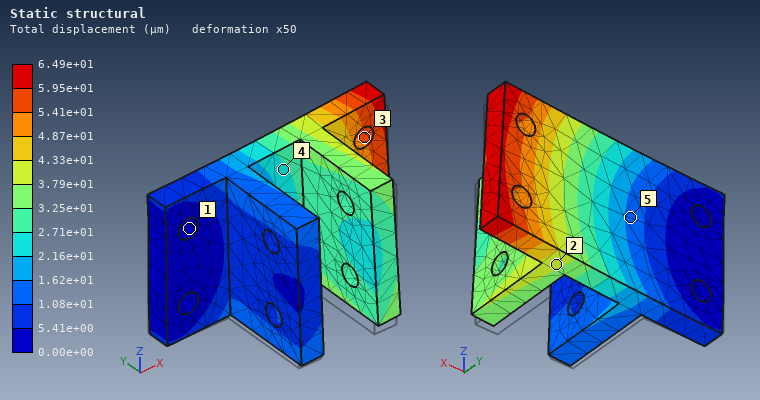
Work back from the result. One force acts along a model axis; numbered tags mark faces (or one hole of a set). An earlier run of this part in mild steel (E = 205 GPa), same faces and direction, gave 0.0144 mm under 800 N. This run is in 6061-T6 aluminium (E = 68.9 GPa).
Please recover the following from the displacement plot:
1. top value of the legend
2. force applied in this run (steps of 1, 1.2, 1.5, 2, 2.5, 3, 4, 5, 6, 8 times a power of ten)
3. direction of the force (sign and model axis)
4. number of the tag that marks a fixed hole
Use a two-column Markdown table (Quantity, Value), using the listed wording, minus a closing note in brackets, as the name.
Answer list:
| Quantity | Value |
|---|---|
| top value of the legend | 6.49e+01 µm |
| force applied in this run | 1.2 kN |
| direction of the force | +Z |
| number of the tag that marks a fixed hole | 1 |
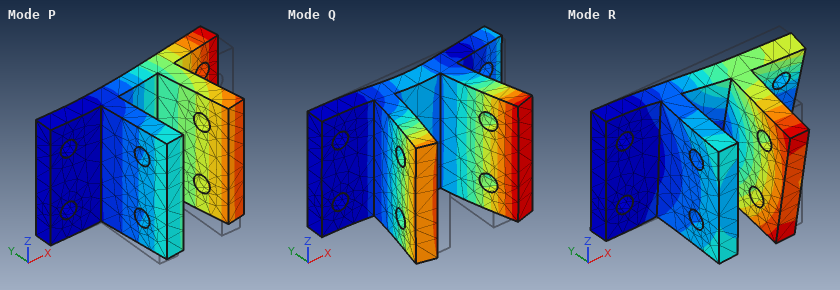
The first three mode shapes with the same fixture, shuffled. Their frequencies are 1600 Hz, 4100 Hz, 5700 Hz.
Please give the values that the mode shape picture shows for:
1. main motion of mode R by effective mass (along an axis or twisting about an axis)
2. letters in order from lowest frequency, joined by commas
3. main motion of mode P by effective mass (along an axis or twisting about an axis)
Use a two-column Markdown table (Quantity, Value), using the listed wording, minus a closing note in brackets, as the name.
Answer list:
| Quantity | Value |
|---|---|
| main motion of mode R by effective mass | along Z |
| letters in order from lowest frequency, joined by commas | P, R, Q |
| main motion of mode P by effective mass | along Y |
